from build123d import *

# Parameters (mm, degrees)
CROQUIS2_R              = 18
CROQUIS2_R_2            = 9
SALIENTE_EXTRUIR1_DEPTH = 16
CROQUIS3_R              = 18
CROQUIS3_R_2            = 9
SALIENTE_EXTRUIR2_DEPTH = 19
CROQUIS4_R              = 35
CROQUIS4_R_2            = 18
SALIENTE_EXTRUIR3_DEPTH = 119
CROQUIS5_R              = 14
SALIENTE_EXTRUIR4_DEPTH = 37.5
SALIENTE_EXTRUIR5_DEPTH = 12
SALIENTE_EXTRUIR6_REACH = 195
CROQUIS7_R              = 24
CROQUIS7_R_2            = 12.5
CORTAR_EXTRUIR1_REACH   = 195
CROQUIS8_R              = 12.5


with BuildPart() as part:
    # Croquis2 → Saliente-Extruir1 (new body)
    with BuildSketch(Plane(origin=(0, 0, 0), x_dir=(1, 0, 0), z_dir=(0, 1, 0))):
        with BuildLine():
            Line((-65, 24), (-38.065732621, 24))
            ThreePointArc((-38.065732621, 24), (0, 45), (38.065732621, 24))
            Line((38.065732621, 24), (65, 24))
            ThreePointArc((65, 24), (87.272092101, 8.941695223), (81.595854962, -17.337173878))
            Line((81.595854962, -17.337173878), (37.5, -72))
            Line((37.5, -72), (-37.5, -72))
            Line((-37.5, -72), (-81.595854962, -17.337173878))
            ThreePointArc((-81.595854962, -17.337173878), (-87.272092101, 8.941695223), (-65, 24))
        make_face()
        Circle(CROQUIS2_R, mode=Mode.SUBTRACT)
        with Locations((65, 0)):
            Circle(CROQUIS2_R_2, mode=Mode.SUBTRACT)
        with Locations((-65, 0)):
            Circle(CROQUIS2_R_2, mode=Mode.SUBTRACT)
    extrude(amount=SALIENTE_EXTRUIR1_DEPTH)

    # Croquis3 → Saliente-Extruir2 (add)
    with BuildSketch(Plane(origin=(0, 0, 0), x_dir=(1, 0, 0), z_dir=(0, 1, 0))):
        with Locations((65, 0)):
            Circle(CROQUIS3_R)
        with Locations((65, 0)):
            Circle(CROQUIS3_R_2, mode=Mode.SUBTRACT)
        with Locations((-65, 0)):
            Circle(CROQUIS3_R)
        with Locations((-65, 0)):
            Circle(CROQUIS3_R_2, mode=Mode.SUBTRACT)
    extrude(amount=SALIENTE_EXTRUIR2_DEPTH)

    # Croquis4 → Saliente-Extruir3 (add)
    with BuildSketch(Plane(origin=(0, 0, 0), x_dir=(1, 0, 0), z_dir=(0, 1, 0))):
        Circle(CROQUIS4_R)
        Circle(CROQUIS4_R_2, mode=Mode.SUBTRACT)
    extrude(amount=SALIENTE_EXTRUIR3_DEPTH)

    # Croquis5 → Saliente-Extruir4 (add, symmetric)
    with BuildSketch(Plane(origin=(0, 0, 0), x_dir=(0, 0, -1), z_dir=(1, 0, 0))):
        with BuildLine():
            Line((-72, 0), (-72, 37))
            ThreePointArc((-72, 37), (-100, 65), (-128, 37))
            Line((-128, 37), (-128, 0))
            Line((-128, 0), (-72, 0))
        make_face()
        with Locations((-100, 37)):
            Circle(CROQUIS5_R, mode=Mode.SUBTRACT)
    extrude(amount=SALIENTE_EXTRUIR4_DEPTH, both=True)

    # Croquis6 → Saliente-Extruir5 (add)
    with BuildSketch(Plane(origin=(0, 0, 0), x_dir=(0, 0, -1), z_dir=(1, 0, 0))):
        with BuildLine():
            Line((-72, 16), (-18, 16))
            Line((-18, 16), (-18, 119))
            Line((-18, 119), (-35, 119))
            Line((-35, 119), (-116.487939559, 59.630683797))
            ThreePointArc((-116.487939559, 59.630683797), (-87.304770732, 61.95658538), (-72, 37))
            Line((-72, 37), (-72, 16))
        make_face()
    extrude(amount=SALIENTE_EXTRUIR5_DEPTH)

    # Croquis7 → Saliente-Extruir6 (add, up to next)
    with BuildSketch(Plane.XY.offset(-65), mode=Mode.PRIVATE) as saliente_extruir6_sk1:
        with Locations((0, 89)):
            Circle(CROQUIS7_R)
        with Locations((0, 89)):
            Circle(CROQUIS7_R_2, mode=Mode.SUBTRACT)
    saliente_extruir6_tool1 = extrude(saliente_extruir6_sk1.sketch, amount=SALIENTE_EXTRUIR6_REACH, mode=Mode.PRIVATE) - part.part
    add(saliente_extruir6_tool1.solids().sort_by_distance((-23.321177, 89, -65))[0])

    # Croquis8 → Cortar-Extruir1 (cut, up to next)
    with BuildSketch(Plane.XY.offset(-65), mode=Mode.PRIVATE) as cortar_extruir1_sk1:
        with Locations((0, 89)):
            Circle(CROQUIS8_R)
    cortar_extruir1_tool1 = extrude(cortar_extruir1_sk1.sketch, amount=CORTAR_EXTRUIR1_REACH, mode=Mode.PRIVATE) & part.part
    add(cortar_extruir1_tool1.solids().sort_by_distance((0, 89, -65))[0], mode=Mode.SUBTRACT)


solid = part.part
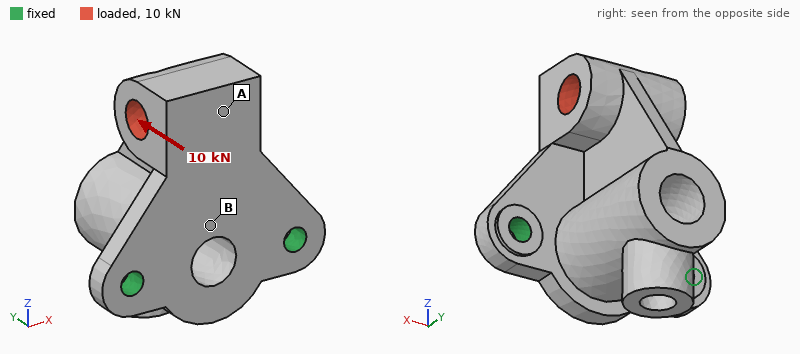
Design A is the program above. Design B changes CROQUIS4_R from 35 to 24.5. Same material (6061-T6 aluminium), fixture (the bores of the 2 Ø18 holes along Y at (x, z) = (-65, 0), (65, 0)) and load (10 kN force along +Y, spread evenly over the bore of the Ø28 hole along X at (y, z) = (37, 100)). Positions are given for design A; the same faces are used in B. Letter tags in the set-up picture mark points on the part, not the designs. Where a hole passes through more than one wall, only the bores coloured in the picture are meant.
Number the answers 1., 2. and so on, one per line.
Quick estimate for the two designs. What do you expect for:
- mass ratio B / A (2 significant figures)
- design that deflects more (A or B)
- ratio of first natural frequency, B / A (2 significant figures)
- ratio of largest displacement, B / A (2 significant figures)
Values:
1. 0.79
2. B
3. 0.99
4. 1.2
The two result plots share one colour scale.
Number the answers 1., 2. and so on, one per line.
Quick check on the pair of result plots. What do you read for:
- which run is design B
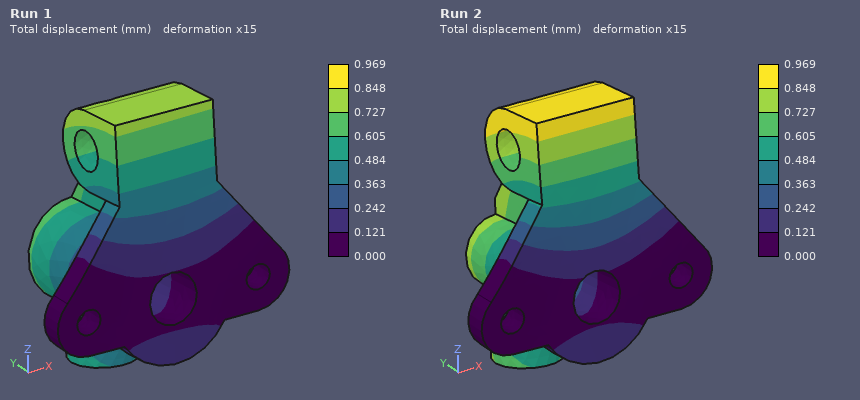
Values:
1. Run 2
